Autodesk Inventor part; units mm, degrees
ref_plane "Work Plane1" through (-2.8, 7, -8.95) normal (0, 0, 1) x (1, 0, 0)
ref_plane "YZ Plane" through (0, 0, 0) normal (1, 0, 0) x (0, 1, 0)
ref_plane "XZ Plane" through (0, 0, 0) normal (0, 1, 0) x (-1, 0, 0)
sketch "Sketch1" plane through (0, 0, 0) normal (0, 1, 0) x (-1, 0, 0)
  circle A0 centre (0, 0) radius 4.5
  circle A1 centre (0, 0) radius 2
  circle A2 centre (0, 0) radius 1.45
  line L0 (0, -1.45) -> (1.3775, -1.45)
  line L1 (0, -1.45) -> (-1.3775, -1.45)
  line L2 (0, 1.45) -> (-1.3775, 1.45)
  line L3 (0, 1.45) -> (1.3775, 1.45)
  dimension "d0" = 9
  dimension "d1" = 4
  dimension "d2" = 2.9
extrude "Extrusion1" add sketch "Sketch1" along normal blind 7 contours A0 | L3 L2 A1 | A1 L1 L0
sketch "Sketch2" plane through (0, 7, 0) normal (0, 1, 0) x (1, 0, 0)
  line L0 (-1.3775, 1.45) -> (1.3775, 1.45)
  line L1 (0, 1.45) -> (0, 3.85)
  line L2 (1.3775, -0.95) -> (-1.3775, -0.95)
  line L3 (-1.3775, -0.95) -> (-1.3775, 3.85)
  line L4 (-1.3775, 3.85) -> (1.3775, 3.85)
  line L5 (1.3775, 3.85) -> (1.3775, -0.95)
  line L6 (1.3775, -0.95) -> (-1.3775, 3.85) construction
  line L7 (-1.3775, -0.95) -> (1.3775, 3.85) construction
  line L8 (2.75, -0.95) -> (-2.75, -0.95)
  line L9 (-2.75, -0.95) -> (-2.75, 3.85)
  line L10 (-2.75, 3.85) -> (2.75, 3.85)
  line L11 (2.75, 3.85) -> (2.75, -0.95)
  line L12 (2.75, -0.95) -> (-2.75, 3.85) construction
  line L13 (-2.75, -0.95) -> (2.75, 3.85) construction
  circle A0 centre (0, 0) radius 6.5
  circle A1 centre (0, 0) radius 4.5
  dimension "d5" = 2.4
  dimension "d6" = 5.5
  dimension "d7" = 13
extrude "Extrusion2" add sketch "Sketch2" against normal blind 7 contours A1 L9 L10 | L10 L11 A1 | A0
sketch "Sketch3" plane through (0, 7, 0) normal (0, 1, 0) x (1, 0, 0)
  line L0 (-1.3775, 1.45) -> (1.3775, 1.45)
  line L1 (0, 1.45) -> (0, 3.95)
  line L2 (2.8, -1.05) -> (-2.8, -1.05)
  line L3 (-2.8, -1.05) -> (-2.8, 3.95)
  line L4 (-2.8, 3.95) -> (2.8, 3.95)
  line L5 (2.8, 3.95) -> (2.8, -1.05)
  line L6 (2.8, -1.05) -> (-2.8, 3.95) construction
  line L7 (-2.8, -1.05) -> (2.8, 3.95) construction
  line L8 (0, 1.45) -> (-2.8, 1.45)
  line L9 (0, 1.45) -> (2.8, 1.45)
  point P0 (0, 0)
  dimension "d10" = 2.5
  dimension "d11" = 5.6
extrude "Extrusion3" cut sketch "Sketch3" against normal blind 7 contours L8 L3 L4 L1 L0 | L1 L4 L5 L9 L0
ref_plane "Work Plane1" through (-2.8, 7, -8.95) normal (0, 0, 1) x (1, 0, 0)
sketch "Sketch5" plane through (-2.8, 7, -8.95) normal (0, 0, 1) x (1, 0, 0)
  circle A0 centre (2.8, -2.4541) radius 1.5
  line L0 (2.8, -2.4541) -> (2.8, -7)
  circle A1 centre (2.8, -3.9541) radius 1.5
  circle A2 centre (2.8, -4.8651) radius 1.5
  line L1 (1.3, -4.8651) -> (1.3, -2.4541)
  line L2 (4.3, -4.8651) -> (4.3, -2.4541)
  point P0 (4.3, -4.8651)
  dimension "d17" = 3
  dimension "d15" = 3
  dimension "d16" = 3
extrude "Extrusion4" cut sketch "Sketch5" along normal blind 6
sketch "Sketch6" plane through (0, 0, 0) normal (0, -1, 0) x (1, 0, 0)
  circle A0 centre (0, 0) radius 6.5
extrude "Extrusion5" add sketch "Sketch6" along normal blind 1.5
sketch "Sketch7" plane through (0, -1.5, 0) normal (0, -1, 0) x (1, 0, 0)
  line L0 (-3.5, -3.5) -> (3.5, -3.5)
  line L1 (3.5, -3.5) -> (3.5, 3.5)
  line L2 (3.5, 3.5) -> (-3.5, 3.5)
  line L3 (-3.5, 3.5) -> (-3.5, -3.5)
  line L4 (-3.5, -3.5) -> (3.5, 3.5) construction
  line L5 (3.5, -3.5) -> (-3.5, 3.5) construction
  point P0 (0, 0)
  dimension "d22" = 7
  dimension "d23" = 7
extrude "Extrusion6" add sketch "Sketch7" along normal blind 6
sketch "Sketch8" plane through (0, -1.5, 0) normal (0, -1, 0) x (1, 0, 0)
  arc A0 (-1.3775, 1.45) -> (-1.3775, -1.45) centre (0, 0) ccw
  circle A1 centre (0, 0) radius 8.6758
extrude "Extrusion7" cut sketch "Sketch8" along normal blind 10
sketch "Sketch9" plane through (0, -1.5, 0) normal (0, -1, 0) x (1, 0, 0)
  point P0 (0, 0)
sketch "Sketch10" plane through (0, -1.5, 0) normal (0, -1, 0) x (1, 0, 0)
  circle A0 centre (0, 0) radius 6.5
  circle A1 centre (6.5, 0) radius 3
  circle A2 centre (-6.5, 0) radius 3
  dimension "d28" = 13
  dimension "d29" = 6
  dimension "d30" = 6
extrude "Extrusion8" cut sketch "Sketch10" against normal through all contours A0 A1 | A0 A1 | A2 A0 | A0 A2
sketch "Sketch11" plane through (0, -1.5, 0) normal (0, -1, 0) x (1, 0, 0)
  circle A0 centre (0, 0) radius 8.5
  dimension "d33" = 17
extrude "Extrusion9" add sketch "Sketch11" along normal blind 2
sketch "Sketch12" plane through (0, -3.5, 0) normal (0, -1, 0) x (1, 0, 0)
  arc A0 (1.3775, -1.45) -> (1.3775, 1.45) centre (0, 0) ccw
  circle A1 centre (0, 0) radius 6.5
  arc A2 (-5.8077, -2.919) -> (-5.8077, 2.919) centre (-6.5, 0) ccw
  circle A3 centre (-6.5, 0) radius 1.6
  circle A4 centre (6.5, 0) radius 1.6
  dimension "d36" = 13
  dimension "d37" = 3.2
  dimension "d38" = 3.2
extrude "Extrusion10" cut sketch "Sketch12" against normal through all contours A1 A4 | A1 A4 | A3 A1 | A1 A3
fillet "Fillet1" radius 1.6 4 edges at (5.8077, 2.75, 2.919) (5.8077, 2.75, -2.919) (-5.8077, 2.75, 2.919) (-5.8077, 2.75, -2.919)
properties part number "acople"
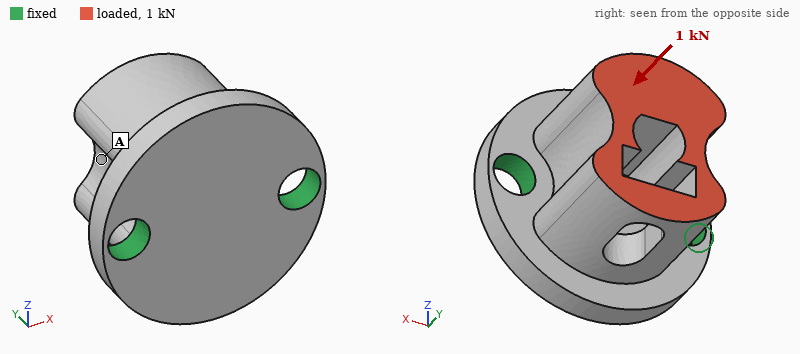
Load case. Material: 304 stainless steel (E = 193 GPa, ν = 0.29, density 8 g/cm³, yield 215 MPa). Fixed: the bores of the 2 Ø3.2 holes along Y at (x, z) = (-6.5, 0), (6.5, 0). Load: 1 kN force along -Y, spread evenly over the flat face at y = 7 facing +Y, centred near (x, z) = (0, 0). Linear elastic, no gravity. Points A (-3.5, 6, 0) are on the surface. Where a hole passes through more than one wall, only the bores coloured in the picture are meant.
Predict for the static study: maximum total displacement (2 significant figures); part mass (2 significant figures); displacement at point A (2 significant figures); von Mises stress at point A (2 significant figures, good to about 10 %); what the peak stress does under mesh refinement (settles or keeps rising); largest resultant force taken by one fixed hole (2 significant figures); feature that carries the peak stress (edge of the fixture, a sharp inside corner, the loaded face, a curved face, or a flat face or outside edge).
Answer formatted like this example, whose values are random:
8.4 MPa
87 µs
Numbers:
4.0 µm
8.8 g
2.7 µm
23 MPa
keeps rising
530 N
edge of the fixture
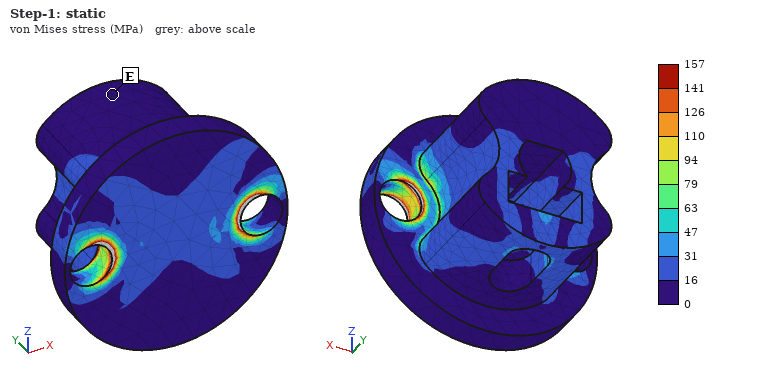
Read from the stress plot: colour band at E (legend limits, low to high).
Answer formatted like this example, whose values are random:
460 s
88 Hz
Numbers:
0 to 16 MPa
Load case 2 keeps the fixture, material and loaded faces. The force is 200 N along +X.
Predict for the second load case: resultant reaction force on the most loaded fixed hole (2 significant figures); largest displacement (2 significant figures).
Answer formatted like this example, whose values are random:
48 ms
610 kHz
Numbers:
210 N
3.0 µm
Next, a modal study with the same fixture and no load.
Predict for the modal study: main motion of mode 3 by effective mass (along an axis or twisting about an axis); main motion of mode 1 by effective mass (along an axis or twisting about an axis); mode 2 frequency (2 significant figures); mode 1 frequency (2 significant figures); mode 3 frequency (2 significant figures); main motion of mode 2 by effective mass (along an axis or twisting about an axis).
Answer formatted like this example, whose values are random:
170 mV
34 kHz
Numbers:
along Y
along Z
32 kHz
15 kHz
39 kHz
along X
